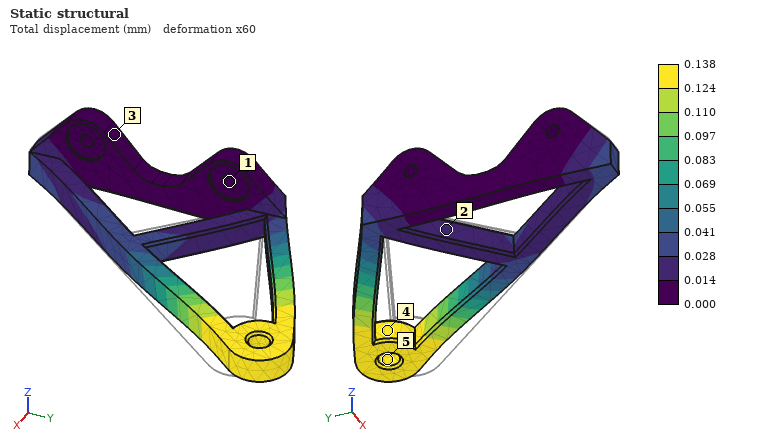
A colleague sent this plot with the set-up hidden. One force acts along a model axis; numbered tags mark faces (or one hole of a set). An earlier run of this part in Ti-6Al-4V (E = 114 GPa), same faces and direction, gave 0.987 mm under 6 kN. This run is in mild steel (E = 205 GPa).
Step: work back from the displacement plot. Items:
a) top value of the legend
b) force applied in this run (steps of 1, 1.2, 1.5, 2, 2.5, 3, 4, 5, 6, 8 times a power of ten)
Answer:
0.138 mm
1.5 kN
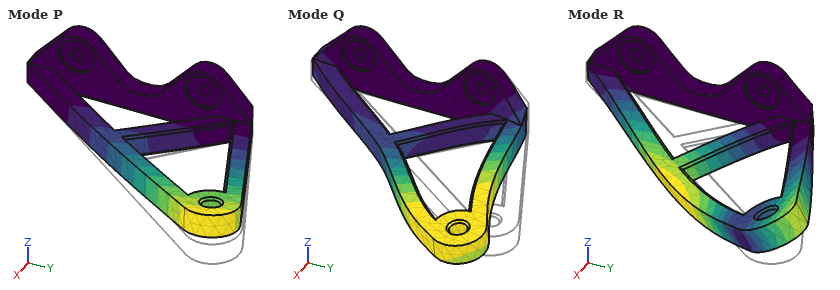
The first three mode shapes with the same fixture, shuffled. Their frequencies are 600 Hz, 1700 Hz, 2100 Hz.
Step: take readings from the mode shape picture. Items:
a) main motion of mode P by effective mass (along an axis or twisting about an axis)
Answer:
along Z
